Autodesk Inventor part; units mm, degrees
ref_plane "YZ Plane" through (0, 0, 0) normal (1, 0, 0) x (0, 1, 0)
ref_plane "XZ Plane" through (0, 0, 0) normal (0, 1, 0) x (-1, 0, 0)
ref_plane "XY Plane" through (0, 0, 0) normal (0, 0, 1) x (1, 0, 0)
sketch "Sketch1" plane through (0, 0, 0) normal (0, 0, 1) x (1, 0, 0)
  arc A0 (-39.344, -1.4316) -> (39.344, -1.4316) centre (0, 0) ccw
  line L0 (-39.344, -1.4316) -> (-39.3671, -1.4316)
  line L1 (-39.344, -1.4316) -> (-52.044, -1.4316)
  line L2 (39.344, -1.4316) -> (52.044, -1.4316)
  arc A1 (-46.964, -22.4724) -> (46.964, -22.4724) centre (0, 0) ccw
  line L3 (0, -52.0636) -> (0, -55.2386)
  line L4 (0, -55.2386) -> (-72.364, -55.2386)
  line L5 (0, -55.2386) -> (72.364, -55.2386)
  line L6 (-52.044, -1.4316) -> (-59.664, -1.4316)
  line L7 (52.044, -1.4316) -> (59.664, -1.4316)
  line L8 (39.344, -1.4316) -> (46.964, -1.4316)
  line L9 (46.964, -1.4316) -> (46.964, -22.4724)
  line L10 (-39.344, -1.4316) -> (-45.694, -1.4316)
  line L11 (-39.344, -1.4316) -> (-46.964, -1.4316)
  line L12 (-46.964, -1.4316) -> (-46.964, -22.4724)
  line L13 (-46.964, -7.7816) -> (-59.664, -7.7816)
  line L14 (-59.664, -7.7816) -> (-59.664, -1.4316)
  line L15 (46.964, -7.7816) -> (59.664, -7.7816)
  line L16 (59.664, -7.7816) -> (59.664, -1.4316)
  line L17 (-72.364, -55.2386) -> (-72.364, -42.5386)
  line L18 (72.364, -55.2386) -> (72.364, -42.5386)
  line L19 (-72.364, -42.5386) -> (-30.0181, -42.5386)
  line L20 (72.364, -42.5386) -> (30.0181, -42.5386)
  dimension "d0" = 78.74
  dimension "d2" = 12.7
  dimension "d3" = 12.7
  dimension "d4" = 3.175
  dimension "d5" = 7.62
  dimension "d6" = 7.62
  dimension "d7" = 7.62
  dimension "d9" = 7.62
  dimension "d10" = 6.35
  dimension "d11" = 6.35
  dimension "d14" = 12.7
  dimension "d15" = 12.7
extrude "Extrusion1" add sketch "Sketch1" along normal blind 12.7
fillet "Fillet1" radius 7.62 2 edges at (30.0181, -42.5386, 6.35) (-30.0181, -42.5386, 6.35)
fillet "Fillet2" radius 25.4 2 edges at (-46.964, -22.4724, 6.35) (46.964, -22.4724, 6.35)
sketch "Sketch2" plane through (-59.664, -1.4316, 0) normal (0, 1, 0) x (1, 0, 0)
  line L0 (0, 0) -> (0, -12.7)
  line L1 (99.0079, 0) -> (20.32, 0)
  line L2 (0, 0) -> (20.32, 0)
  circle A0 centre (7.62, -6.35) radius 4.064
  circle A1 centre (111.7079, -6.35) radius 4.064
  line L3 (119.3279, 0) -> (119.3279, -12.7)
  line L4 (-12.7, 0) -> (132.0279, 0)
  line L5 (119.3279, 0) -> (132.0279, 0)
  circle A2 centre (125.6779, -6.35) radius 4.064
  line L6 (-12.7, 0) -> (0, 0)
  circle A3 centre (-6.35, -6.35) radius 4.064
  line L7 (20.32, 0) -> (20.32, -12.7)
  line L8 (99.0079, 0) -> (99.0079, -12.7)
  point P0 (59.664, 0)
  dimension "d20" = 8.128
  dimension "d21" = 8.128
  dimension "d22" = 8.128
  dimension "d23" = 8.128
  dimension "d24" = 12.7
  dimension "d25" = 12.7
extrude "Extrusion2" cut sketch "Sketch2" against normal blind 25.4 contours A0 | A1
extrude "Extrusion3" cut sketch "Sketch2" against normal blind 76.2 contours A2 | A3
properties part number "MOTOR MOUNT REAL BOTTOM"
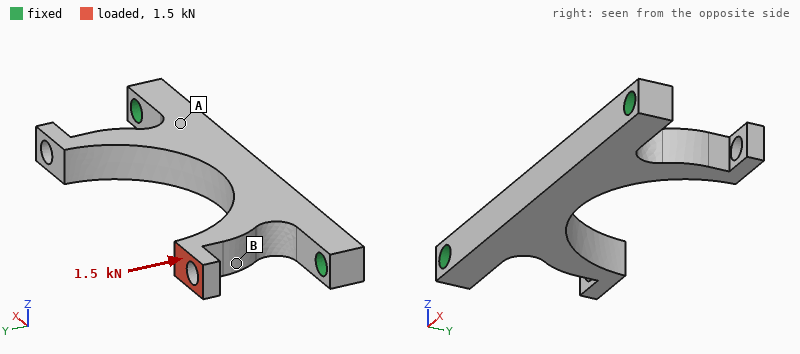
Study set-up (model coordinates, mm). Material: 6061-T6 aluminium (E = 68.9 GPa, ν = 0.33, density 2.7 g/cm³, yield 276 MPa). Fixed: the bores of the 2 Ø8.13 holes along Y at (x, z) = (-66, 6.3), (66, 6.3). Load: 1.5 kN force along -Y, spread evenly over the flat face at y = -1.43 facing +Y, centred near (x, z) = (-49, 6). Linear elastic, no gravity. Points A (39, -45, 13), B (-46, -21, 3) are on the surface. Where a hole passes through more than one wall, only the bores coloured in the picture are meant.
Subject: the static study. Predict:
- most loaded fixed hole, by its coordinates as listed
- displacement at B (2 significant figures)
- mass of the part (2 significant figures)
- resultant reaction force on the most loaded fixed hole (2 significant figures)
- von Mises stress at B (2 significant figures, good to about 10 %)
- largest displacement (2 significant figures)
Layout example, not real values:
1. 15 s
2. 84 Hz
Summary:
1. (-66, 6.3)
2. 0.050 mm
3. 110 g
4. 1.5 kN
5. 44 MPa
6. 0.20 mm
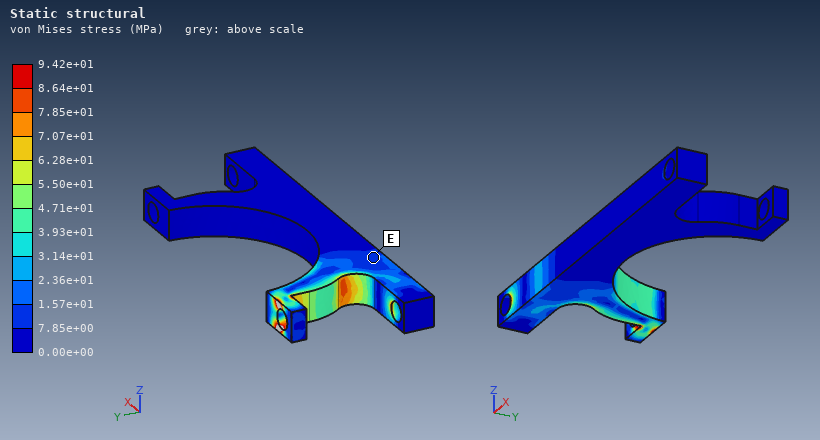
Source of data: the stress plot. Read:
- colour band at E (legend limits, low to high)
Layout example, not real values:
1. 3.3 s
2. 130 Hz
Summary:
1. 7.85e+00 to 1.57e+01 MPa
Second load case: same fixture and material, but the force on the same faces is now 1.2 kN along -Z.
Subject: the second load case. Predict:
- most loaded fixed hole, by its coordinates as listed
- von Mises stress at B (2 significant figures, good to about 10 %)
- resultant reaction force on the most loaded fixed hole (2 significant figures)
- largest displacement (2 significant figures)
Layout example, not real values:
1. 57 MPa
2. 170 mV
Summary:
1. (-66, 6.3)
2. 36 MPa
3. 1.2 kN
4. 0.79 mm
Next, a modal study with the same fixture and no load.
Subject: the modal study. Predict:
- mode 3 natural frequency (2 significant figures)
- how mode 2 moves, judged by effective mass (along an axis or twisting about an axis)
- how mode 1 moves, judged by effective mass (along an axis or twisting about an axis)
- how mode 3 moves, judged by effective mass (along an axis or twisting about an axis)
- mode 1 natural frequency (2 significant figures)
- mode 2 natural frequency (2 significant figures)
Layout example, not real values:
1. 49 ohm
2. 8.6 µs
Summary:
1. 3300 Hz
2. twisting about Y
3. along Z
4. along Y
5. 2100 Hz
6. 3100 Hz
